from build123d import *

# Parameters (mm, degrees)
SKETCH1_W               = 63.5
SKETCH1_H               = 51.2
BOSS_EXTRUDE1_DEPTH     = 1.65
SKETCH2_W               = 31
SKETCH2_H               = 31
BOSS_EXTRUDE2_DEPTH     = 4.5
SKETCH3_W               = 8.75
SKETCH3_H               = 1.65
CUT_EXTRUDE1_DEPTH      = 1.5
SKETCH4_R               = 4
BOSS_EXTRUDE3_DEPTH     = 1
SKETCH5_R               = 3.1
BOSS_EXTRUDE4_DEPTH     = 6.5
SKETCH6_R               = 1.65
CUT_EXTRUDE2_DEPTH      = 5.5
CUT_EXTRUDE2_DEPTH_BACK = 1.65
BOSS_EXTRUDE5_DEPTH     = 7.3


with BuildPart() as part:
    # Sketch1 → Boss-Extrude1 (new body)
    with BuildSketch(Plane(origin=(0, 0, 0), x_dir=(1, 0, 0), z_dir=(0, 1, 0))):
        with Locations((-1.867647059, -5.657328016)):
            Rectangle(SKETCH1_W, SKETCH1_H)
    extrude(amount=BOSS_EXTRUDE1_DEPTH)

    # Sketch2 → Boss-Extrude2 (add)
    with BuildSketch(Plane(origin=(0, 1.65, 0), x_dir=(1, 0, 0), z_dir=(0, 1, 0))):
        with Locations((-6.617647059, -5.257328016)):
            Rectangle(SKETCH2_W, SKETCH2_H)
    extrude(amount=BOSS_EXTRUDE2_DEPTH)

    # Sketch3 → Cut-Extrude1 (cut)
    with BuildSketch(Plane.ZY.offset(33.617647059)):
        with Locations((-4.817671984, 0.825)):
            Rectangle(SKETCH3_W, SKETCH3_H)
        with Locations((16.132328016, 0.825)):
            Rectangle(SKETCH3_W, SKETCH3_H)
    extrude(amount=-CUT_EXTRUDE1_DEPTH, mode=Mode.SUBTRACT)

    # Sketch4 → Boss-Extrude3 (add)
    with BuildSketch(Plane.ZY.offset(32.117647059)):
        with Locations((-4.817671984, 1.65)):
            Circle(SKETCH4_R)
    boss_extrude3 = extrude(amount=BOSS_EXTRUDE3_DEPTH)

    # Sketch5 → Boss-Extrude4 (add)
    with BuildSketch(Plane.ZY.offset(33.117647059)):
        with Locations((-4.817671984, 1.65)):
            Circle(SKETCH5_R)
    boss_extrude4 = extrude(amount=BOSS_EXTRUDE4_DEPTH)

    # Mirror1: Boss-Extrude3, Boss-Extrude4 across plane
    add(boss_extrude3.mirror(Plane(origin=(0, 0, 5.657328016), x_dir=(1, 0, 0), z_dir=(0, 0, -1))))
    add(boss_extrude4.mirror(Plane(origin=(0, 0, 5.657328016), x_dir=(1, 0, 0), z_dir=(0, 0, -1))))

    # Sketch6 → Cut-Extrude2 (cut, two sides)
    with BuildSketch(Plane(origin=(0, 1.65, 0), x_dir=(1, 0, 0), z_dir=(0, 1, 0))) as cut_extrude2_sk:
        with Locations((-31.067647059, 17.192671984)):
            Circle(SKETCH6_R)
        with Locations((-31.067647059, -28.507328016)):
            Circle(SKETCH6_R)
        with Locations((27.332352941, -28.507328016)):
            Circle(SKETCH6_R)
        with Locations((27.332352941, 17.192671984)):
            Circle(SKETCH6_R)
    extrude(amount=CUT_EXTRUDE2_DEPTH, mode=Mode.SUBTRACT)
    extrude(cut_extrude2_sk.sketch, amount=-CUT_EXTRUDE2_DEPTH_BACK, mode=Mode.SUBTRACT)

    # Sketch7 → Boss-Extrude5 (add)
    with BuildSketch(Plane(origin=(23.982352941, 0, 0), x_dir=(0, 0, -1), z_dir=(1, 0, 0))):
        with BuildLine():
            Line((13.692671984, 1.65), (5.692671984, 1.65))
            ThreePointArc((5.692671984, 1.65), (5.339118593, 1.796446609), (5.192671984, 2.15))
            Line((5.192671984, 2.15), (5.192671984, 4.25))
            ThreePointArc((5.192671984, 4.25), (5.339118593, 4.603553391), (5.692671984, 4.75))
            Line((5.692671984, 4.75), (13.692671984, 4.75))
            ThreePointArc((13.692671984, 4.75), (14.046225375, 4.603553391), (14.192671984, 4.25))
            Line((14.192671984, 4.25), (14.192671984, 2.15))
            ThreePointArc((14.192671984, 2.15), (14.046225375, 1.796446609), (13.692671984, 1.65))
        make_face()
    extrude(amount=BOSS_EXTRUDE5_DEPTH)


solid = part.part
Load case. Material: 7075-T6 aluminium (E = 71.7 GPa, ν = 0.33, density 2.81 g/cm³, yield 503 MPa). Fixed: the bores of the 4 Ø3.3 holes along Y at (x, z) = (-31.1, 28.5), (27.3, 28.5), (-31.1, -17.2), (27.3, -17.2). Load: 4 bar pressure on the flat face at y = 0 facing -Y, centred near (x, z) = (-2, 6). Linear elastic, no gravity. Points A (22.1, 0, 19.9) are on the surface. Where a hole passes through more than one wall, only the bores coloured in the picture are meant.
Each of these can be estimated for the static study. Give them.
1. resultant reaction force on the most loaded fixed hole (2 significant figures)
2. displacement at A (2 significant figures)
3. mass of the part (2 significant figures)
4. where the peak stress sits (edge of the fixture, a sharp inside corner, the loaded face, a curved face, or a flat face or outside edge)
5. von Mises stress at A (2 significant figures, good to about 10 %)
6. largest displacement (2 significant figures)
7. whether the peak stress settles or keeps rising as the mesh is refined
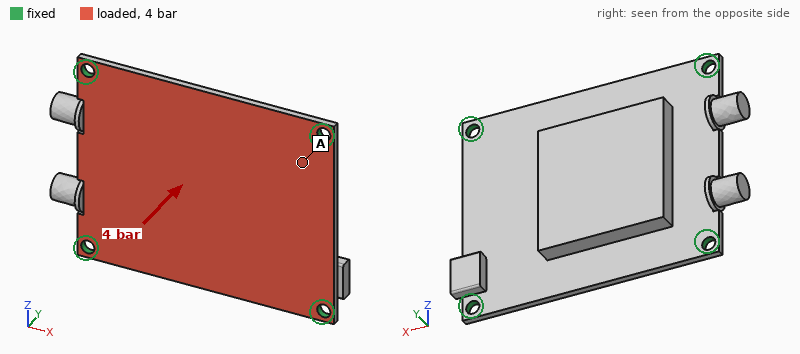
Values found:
360 N
0.15 mm
29 g
edge of the fixture
57 MPa
0.33 mm
keeps rising
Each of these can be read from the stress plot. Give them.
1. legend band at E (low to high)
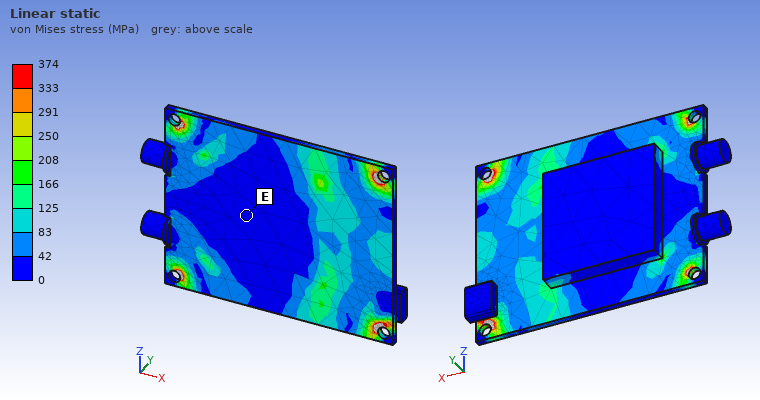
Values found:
0 to 42 MPa
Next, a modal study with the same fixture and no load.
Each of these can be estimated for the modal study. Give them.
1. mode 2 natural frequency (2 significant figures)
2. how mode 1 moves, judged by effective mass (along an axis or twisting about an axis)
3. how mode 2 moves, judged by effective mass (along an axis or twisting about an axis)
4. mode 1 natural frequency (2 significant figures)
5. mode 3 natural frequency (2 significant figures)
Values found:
3900 Hz
along Y
twisting about X
2100 Hz
4100 Hz
